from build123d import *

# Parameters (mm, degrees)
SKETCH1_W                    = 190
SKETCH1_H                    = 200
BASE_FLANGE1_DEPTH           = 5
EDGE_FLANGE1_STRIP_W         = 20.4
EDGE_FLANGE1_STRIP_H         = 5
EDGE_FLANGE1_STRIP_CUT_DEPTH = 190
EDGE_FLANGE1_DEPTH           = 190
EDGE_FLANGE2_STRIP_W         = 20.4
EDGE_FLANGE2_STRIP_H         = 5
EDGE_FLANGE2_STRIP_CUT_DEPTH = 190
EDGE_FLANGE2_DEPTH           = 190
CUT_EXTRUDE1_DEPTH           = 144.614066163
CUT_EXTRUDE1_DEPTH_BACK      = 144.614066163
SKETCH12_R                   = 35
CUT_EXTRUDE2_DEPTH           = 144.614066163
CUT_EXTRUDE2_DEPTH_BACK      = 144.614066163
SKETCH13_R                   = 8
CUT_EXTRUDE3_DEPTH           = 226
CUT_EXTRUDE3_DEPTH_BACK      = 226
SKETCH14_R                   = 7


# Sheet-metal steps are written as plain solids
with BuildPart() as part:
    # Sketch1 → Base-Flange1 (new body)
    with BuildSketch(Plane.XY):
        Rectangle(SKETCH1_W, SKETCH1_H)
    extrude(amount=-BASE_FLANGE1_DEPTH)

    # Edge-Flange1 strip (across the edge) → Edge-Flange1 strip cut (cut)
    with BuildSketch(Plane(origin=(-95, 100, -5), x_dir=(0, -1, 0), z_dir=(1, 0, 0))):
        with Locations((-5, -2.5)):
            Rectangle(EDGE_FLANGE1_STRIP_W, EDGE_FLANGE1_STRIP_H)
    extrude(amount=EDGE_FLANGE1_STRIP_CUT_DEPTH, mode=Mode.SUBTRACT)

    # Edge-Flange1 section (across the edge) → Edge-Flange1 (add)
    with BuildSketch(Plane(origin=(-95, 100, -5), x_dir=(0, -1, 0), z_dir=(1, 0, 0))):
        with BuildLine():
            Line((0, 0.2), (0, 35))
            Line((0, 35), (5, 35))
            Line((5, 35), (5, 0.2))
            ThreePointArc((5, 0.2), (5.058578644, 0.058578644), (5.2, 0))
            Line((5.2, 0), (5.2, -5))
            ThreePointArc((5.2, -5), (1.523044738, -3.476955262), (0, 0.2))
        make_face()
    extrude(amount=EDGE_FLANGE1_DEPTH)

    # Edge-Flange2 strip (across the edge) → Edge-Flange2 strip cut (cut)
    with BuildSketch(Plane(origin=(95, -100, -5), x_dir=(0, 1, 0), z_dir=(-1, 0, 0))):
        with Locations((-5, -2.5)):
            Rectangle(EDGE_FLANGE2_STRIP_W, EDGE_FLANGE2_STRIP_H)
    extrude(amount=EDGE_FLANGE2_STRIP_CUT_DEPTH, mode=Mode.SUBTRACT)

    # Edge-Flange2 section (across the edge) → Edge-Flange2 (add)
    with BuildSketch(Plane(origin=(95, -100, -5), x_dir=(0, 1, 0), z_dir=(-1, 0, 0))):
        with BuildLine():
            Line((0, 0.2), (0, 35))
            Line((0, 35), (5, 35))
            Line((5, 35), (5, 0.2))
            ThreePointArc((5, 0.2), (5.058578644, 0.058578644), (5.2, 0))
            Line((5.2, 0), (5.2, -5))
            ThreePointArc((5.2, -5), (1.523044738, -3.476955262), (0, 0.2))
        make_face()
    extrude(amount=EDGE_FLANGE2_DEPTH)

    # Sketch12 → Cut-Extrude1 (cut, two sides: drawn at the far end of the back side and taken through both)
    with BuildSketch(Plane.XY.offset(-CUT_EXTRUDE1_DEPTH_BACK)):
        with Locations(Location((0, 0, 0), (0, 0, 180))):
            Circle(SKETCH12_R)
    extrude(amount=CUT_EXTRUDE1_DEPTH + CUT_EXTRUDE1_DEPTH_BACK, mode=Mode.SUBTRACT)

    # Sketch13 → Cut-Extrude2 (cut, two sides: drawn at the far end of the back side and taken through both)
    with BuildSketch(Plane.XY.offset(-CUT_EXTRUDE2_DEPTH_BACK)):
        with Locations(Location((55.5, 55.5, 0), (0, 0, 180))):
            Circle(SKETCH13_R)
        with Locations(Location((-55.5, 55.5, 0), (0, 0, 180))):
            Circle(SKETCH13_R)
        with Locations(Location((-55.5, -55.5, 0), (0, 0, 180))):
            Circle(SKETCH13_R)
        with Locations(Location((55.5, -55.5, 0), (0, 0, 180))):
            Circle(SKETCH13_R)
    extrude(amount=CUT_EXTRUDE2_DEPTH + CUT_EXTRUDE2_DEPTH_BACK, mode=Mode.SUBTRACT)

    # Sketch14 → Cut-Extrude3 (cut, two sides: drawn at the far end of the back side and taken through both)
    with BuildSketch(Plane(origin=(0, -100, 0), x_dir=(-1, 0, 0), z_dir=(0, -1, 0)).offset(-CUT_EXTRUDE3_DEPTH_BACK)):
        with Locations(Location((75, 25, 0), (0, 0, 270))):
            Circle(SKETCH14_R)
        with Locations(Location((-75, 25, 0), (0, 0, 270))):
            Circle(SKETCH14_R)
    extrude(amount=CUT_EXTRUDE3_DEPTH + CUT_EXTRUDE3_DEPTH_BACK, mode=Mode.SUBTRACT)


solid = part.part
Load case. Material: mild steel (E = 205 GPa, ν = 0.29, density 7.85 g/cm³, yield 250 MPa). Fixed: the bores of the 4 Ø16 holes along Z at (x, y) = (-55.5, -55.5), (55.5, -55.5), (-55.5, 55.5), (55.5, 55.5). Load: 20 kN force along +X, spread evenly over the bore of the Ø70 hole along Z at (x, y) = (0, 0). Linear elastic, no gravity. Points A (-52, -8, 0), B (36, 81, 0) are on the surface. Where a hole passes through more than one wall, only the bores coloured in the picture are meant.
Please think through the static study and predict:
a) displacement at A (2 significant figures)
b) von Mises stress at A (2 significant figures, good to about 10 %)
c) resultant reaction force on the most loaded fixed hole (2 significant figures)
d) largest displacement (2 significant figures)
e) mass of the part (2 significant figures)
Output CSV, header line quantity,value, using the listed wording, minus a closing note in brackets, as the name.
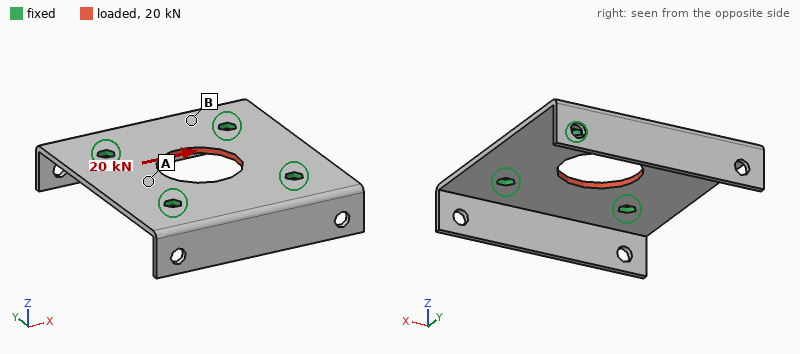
quantity,value
displacement at A,6.4 µm
von Mises stress at A,13 MPa
resultant reaction force on the most loaded fixed hole,5.2 kN
largest displacement,7.9 µm
mass of the part,1.8 kg
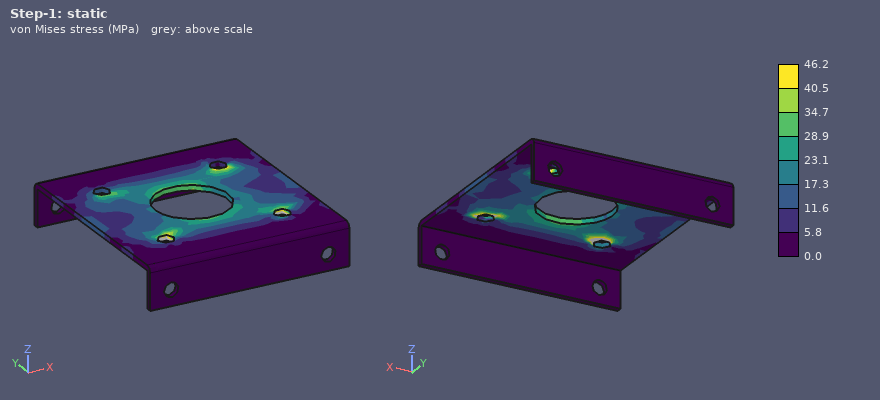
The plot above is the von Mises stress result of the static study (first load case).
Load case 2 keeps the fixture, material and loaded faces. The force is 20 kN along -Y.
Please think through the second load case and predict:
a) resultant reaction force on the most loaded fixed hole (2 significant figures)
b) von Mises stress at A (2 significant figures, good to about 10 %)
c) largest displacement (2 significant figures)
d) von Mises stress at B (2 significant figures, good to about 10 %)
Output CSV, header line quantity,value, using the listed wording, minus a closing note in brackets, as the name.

quantity,value
resultant reaction force on the most loaded fixed hole,5.1 kN
von Mises stress at A,15 MPa
largest displacement,7.4 µm
von Mises stress at B,11 MPa
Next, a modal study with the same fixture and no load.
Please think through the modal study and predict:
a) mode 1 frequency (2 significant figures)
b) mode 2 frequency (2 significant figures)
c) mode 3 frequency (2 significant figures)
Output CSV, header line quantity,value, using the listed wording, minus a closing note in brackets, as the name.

quantity,value
mode 1 frequency,930 Hz
mode 2 frequency,930 Hz
mode 3 frequency,1200 Hz
